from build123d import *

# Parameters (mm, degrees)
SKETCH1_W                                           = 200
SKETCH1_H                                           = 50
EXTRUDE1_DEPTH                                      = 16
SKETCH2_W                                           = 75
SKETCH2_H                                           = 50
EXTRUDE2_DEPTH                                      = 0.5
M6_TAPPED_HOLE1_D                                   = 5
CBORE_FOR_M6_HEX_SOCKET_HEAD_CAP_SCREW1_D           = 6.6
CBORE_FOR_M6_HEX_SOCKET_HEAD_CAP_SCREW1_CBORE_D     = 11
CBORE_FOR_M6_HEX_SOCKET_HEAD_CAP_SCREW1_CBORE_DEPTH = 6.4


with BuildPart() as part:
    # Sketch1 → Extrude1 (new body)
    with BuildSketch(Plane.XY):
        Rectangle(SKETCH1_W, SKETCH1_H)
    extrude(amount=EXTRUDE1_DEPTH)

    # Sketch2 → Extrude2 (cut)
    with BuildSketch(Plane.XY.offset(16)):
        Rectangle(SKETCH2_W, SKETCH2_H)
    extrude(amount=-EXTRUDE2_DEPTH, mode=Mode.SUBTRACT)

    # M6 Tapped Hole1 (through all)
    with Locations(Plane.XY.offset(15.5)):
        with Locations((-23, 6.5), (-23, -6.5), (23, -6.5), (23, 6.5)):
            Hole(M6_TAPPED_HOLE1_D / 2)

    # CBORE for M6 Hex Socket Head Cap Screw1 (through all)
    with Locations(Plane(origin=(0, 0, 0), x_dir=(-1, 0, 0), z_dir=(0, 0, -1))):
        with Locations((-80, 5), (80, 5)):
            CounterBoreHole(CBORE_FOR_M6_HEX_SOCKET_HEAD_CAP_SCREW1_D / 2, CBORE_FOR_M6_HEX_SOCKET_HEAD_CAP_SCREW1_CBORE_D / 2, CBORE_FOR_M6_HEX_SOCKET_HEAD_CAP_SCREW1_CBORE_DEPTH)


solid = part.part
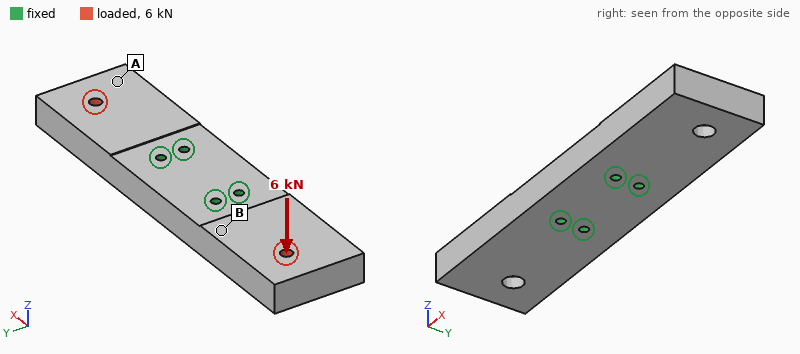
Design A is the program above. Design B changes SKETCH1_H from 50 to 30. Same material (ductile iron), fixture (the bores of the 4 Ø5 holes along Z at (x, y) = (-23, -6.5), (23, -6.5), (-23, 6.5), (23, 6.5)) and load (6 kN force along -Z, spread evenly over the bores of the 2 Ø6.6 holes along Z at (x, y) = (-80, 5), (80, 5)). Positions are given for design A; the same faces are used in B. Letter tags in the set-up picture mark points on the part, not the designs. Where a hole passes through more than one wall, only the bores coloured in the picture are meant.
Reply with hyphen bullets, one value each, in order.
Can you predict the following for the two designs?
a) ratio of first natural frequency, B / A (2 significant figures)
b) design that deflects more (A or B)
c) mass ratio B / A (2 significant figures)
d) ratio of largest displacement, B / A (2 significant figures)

- 1.1
- B
- 0.59
- 1.5
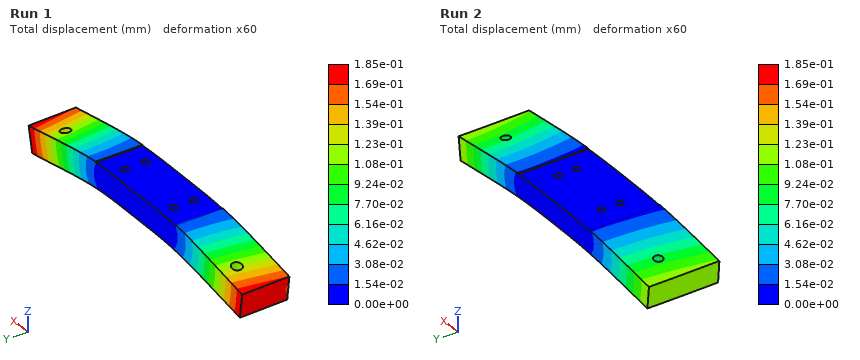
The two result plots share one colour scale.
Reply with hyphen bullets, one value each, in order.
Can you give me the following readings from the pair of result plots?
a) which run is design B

- Run 1
